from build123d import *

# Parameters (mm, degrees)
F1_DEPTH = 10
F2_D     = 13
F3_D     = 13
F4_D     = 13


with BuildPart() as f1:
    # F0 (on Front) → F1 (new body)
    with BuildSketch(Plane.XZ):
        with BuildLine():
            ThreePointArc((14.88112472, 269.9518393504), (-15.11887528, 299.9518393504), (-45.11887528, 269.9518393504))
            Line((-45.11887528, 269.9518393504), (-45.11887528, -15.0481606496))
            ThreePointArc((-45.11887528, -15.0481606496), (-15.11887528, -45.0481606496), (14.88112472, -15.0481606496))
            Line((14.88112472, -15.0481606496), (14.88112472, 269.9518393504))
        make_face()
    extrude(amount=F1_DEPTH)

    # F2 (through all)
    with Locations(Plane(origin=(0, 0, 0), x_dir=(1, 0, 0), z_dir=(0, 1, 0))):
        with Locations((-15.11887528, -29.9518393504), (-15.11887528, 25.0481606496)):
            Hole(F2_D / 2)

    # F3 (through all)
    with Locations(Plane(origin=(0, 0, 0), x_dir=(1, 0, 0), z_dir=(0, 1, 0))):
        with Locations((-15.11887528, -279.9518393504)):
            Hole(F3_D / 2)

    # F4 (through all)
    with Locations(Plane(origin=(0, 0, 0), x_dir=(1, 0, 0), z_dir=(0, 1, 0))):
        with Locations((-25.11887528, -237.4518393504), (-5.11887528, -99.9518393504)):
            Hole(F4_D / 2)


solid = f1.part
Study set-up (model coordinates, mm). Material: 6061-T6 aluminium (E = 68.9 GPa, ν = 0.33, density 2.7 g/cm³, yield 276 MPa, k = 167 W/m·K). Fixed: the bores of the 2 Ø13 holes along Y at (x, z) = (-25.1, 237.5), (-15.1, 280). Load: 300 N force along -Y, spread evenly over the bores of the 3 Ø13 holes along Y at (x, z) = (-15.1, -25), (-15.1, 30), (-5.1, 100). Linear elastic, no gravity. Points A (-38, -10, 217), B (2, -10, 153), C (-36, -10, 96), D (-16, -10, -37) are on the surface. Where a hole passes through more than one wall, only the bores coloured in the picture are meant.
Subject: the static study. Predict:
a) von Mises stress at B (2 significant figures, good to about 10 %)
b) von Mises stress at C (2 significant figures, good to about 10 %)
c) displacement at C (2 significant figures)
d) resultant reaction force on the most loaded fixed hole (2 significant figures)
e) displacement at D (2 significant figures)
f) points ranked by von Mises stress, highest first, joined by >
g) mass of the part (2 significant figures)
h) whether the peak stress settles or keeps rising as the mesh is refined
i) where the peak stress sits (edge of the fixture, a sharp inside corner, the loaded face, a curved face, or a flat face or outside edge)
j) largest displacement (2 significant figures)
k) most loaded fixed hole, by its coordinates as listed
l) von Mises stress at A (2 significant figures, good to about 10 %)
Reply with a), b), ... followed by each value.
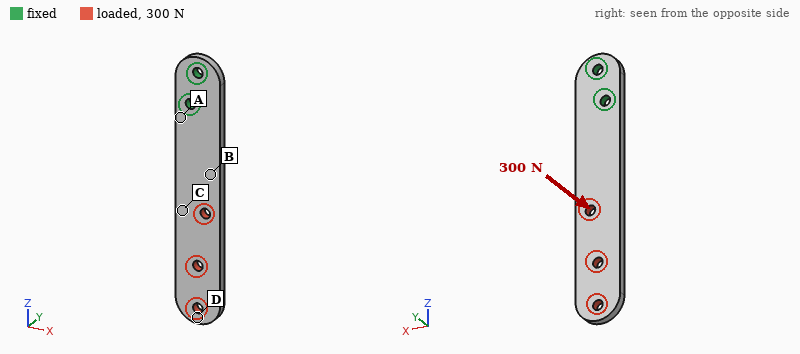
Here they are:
a) 35 MPa
b) 22 MPa
c) 1.3 mm
d) 720 N
e) 3.7 mm
f) A > B > C > D
g) 520 g
h) keeps rising
i) edge of the fixture
j) 3.9 mm
k) (-25.1, 237.5)
l) 57 MPa
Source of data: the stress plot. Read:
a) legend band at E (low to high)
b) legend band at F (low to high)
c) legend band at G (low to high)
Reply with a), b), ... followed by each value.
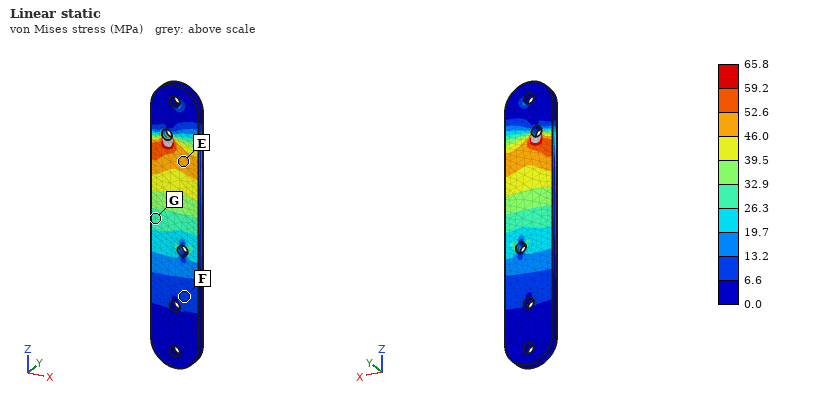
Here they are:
a) 46.0 to 52.6 MPa
b) 6.6 to 13.2 MPa
c) 26.3 to 32.9 MPa
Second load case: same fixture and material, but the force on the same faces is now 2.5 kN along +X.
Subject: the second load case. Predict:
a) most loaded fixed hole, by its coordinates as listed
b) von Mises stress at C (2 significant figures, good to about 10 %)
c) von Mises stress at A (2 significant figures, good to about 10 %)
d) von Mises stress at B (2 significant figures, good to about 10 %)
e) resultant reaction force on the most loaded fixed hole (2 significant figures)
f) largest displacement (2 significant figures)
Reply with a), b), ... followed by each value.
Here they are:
a) (-25.1, 237.5)
b) 19 MPa
c) 58 MPa
d) 30 MPa
e) 11 kN
f) 1.2 mm
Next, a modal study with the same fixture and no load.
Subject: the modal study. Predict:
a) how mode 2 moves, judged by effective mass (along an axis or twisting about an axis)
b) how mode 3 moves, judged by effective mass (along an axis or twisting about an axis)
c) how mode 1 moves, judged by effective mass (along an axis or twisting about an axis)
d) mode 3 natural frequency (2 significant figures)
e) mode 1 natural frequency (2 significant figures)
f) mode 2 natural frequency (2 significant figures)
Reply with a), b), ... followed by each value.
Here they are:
a) along X
b) along Y
c) along Y
d) 670 Hz
e) 110 Hz
f) 550 Hz
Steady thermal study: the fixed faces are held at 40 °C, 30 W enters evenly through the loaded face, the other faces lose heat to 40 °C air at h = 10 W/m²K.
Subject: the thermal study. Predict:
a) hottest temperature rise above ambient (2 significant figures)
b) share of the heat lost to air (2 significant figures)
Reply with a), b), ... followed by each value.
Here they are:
a) 46 K
b) 34 %
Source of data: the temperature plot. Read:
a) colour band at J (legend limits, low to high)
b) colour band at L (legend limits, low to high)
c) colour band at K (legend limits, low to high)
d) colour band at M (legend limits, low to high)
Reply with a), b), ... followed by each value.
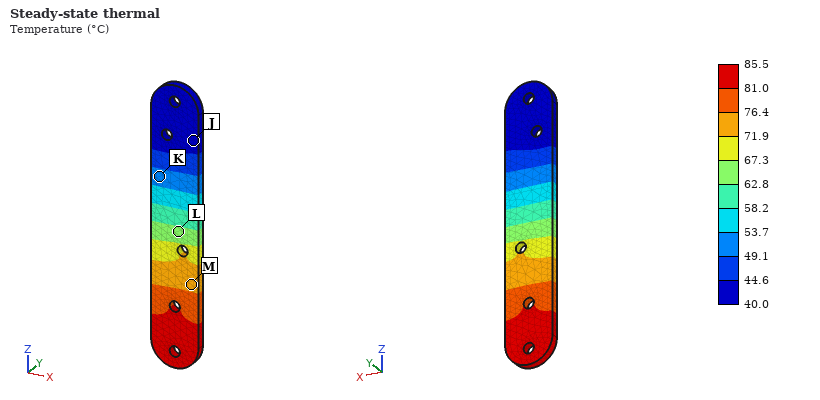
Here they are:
a) 40.0 to 44.6 °C
b) 62.8 to 67.3 °C
c) 49.1 to 53.7 °C
d) 71.9 to 76.4 °C
